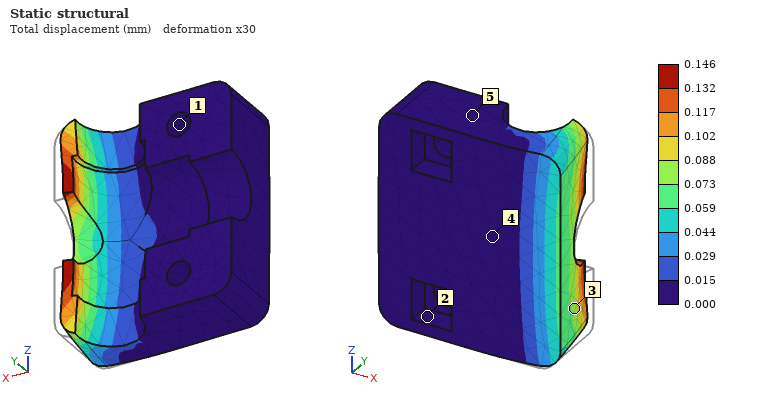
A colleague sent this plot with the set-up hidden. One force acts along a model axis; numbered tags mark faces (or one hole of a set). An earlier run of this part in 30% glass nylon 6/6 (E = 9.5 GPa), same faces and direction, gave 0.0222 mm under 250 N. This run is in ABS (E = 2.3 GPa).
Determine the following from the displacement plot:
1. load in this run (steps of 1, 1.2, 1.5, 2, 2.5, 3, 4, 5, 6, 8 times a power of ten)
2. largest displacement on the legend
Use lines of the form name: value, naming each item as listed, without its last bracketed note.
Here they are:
load in this run: 400 N
largest displacement on the legend: 0.146 mm
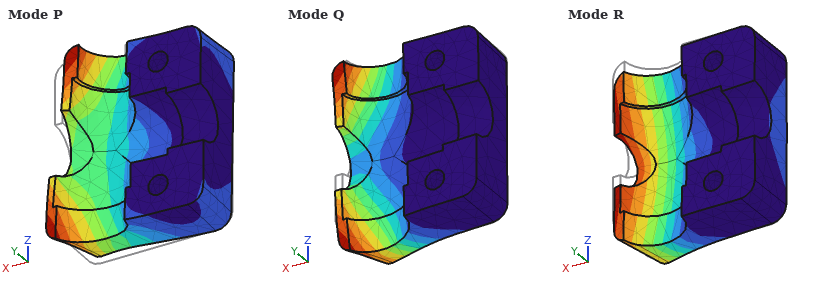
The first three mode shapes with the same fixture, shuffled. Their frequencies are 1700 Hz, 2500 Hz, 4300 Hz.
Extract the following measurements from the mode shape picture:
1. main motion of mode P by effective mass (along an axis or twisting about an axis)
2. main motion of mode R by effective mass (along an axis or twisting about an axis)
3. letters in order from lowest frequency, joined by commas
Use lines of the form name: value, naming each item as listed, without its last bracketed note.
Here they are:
main motion of mode P by effective mass: along Z
main motion of mode R by effective mass: along Y
letters in order from lowest frequency, joined by commas: R, Q, P
